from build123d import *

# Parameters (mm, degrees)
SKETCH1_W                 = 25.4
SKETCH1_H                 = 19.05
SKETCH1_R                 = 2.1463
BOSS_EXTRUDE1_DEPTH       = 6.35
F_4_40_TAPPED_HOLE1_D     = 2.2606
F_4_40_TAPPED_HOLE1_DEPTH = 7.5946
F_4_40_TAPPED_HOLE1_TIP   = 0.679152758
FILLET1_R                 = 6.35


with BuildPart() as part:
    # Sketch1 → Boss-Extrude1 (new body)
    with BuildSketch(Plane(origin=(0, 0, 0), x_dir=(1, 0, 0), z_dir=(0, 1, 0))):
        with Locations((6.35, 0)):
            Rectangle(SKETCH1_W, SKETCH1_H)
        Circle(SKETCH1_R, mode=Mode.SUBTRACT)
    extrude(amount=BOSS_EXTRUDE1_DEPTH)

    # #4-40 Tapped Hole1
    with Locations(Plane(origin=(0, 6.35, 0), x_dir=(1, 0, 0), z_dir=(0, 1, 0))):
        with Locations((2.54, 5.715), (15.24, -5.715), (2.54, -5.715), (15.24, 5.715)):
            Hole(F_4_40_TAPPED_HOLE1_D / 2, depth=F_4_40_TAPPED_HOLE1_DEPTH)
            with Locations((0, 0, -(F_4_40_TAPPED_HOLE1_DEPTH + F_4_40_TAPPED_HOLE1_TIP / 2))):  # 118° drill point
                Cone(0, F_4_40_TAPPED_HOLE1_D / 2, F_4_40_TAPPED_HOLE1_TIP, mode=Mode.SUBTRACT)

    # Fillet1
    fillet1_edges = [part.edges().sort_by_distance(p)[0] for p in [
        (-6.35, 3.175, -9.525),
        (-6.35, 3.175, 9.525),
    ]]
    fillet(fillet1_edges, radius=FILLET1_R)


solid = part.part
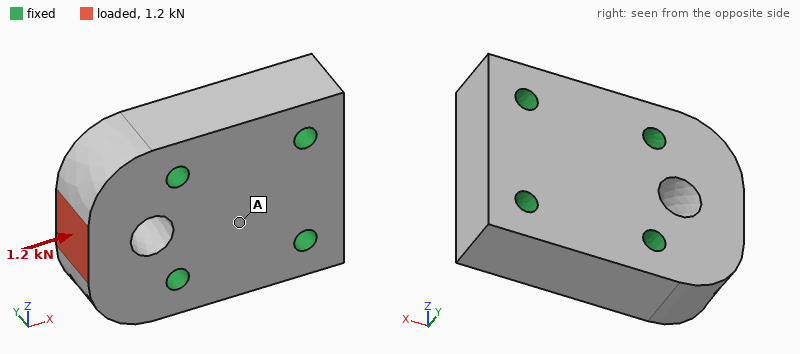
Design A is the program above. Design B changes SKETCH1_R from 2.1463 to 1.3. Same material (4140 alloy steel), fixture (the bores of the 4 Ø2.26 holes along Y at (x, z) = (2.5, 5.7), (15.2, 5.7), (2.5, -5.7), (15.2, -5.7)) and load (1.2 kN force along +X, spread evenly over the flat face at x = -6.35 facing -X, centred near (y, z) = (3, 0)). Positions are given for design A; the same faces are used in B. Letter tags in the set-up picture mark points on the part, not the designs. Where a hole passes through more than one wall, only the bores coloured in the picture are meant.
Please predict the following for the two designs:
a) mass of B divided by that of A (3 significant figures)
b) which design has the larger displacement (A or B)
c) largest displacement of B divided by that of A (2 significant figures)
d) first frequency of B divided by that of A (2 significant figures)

1.02
A
0.84
1.0
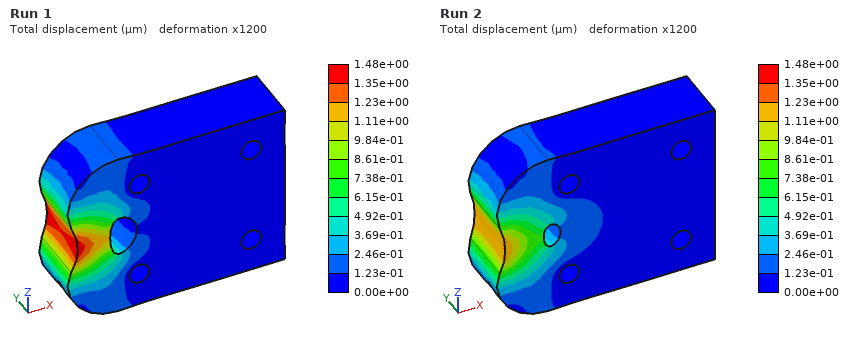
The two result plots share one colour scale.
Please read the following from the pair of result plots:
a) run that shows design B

Run 2
